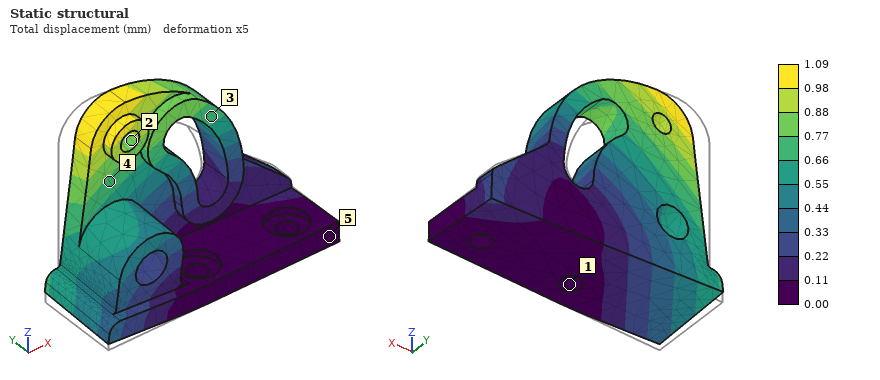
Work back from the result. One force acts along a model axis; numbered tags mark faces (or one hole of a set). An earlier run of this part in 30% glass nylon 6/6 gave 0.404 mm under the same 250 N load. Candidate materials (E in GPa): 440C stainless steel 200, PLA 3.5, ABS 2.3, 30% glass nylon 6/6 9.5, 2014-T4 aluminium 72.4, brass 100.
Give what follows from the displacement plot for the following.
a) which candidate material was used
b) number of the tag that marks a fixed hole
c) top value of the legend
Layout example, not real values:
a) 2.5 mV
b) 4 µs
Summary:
a) PLA
b) 1
c) 1.09 mm
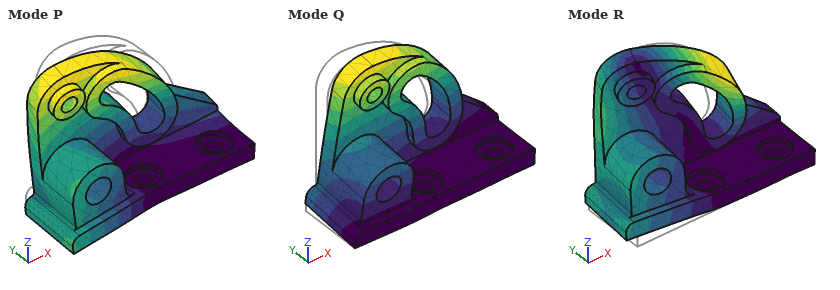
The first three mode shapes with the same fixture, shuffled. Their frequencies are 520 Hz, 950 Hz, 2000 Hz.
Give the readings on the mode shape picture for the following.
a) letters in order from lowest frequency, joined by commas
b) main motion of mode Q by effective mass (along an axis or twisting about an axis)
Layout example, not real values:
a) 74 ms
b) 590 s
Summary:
a) Q, P, R
b) along Y
